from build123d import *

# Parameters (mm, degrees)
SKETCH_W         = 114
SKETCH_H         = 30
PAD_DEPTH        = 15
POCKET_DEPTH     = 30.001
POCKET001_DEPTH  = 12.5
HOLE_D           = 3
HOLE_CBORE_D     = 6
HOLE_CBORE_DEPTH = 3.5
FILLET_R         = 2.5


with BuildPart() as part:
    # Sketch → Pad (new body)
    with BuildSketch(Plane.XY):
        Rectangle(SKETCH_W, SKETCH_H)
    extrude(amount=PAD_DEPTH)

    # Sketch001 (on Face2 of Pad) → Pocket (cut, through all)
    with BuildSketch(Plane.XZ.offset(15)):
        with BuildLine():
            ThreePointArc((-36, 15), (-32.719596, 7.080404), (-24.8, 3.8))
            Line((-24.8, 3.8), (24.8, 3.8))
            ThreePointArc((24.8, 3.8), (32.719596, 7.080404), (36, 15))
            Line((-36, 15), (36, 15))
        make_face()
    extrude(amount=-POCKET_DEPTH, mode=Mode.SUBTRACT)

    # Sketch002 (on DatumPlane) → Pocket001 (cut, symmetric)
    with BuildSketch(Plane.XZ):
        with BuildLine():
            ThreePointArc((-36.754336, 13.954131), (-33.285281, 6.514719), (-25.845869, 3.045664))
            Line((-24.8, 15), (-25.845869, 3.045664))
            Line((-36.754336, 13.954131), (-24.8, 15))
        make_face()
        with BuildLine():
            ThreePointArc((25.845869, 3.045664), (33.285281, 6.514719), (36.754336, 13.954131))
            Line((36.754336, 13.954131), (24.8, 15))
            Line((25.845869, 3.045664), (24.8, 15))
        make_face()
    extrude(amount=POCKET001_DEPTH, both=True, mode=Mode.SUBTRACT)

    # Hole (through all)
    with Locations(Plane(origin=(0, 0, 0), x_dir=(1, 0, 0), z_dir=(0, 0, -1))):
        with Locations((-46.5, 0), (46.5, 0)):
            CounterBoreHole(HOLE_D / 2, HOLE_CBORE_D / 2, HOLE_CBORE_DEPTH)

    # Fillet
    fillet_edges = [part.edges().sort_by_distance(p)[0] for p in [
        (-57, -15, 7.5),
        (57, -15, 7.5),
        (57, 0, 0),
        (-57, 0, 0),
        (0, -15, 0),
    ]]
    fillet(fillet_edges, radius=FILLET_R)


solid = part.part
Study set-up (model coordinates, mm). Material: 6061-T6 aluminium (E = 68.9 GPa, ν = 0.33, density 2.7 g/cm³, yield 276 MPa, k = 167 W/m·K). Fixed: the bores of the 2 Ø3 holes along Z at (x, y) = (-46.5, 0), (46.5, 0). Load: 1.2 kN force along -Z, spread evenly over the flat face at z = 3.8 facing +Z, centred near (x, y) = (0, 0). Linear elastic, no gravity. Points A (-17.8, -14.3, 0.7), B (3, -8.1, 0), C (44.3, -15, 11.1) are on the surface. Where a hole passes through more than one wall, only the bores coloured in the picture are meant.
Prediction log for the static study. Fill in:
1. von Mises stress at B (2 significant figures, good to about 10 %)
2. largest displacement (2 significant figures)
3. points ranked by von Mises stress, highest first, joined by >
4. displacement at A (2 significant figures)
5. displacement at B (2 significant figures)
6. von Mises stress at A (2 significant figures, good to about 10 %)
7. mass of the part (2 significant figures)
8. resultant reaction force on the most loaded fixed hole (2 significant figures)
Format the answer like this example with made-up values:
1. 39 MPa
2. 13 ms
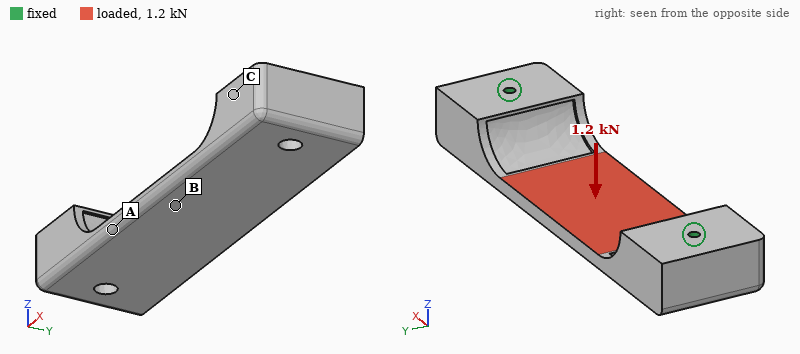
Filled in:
1. 67 MPa
2. 0.15 mm
3. B > A > C
4. 0.077 mm
5. 0.14 mm
6. 25 MPa
7. 74 g
8. 980 N
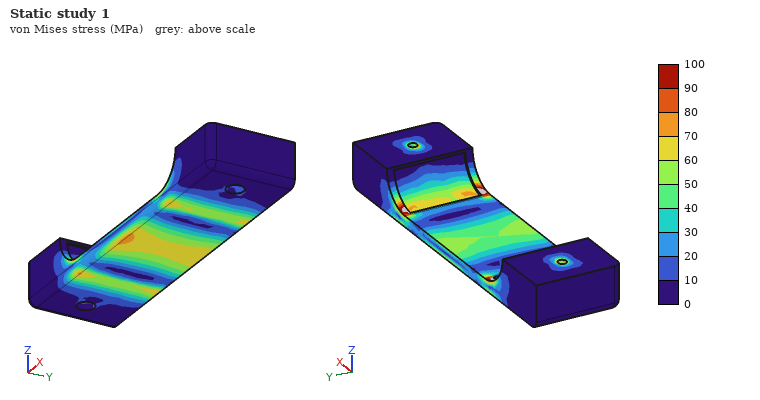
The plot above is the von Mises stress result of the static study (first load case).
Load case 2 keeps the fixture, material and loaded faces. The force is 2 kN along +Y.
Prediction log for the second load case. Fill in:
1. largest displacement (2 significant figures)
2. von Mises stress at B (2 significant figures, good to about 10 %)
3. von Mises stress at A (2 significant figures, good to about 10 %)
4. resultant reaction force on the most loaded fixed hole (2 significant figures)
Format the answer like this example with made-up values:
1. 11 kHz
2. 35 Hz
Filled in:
1. 55 µm
2. 30 MPa
3. 40 MPa
4. 1.0 kN
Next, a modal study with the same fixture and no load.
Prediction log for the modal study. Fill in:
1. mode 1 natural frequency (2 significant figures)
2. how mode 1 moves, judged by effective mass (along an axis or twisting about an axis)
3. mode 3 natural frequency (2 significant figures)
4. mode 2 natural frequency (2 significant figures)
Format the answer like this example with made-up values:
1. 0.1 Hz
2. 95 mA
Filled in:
1. 4300 Hz
2. along Z
3. 7600 Hz
4. 6900 Hz
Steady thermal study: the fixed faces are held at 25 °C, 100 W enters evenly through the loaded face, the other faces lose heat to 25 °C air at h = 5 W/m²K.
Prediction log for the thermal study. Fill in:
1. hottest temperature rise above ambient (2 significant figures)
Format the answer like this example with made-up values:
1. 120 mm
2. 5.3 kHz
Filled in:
1. 74 K
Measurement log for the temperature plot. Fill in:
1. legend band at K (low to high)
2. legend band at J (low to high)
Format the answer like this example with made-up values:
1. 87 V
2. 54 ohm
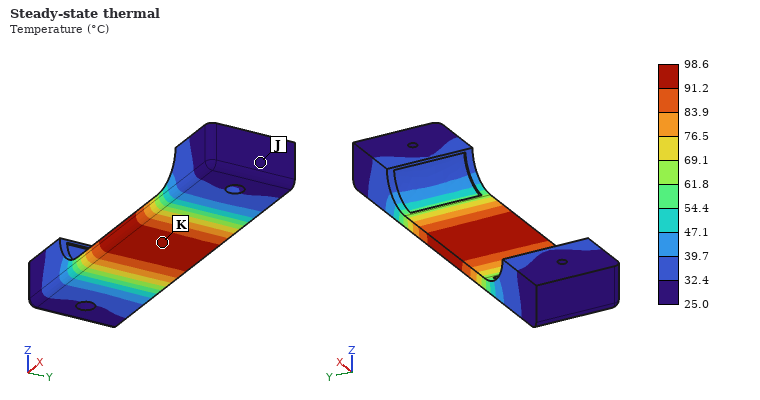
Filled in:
1. 91.2 to 98.6 °C
2. 25.0 to 32.4 °C
